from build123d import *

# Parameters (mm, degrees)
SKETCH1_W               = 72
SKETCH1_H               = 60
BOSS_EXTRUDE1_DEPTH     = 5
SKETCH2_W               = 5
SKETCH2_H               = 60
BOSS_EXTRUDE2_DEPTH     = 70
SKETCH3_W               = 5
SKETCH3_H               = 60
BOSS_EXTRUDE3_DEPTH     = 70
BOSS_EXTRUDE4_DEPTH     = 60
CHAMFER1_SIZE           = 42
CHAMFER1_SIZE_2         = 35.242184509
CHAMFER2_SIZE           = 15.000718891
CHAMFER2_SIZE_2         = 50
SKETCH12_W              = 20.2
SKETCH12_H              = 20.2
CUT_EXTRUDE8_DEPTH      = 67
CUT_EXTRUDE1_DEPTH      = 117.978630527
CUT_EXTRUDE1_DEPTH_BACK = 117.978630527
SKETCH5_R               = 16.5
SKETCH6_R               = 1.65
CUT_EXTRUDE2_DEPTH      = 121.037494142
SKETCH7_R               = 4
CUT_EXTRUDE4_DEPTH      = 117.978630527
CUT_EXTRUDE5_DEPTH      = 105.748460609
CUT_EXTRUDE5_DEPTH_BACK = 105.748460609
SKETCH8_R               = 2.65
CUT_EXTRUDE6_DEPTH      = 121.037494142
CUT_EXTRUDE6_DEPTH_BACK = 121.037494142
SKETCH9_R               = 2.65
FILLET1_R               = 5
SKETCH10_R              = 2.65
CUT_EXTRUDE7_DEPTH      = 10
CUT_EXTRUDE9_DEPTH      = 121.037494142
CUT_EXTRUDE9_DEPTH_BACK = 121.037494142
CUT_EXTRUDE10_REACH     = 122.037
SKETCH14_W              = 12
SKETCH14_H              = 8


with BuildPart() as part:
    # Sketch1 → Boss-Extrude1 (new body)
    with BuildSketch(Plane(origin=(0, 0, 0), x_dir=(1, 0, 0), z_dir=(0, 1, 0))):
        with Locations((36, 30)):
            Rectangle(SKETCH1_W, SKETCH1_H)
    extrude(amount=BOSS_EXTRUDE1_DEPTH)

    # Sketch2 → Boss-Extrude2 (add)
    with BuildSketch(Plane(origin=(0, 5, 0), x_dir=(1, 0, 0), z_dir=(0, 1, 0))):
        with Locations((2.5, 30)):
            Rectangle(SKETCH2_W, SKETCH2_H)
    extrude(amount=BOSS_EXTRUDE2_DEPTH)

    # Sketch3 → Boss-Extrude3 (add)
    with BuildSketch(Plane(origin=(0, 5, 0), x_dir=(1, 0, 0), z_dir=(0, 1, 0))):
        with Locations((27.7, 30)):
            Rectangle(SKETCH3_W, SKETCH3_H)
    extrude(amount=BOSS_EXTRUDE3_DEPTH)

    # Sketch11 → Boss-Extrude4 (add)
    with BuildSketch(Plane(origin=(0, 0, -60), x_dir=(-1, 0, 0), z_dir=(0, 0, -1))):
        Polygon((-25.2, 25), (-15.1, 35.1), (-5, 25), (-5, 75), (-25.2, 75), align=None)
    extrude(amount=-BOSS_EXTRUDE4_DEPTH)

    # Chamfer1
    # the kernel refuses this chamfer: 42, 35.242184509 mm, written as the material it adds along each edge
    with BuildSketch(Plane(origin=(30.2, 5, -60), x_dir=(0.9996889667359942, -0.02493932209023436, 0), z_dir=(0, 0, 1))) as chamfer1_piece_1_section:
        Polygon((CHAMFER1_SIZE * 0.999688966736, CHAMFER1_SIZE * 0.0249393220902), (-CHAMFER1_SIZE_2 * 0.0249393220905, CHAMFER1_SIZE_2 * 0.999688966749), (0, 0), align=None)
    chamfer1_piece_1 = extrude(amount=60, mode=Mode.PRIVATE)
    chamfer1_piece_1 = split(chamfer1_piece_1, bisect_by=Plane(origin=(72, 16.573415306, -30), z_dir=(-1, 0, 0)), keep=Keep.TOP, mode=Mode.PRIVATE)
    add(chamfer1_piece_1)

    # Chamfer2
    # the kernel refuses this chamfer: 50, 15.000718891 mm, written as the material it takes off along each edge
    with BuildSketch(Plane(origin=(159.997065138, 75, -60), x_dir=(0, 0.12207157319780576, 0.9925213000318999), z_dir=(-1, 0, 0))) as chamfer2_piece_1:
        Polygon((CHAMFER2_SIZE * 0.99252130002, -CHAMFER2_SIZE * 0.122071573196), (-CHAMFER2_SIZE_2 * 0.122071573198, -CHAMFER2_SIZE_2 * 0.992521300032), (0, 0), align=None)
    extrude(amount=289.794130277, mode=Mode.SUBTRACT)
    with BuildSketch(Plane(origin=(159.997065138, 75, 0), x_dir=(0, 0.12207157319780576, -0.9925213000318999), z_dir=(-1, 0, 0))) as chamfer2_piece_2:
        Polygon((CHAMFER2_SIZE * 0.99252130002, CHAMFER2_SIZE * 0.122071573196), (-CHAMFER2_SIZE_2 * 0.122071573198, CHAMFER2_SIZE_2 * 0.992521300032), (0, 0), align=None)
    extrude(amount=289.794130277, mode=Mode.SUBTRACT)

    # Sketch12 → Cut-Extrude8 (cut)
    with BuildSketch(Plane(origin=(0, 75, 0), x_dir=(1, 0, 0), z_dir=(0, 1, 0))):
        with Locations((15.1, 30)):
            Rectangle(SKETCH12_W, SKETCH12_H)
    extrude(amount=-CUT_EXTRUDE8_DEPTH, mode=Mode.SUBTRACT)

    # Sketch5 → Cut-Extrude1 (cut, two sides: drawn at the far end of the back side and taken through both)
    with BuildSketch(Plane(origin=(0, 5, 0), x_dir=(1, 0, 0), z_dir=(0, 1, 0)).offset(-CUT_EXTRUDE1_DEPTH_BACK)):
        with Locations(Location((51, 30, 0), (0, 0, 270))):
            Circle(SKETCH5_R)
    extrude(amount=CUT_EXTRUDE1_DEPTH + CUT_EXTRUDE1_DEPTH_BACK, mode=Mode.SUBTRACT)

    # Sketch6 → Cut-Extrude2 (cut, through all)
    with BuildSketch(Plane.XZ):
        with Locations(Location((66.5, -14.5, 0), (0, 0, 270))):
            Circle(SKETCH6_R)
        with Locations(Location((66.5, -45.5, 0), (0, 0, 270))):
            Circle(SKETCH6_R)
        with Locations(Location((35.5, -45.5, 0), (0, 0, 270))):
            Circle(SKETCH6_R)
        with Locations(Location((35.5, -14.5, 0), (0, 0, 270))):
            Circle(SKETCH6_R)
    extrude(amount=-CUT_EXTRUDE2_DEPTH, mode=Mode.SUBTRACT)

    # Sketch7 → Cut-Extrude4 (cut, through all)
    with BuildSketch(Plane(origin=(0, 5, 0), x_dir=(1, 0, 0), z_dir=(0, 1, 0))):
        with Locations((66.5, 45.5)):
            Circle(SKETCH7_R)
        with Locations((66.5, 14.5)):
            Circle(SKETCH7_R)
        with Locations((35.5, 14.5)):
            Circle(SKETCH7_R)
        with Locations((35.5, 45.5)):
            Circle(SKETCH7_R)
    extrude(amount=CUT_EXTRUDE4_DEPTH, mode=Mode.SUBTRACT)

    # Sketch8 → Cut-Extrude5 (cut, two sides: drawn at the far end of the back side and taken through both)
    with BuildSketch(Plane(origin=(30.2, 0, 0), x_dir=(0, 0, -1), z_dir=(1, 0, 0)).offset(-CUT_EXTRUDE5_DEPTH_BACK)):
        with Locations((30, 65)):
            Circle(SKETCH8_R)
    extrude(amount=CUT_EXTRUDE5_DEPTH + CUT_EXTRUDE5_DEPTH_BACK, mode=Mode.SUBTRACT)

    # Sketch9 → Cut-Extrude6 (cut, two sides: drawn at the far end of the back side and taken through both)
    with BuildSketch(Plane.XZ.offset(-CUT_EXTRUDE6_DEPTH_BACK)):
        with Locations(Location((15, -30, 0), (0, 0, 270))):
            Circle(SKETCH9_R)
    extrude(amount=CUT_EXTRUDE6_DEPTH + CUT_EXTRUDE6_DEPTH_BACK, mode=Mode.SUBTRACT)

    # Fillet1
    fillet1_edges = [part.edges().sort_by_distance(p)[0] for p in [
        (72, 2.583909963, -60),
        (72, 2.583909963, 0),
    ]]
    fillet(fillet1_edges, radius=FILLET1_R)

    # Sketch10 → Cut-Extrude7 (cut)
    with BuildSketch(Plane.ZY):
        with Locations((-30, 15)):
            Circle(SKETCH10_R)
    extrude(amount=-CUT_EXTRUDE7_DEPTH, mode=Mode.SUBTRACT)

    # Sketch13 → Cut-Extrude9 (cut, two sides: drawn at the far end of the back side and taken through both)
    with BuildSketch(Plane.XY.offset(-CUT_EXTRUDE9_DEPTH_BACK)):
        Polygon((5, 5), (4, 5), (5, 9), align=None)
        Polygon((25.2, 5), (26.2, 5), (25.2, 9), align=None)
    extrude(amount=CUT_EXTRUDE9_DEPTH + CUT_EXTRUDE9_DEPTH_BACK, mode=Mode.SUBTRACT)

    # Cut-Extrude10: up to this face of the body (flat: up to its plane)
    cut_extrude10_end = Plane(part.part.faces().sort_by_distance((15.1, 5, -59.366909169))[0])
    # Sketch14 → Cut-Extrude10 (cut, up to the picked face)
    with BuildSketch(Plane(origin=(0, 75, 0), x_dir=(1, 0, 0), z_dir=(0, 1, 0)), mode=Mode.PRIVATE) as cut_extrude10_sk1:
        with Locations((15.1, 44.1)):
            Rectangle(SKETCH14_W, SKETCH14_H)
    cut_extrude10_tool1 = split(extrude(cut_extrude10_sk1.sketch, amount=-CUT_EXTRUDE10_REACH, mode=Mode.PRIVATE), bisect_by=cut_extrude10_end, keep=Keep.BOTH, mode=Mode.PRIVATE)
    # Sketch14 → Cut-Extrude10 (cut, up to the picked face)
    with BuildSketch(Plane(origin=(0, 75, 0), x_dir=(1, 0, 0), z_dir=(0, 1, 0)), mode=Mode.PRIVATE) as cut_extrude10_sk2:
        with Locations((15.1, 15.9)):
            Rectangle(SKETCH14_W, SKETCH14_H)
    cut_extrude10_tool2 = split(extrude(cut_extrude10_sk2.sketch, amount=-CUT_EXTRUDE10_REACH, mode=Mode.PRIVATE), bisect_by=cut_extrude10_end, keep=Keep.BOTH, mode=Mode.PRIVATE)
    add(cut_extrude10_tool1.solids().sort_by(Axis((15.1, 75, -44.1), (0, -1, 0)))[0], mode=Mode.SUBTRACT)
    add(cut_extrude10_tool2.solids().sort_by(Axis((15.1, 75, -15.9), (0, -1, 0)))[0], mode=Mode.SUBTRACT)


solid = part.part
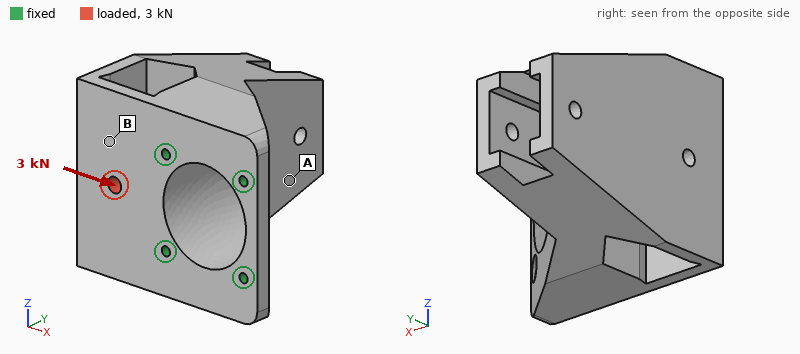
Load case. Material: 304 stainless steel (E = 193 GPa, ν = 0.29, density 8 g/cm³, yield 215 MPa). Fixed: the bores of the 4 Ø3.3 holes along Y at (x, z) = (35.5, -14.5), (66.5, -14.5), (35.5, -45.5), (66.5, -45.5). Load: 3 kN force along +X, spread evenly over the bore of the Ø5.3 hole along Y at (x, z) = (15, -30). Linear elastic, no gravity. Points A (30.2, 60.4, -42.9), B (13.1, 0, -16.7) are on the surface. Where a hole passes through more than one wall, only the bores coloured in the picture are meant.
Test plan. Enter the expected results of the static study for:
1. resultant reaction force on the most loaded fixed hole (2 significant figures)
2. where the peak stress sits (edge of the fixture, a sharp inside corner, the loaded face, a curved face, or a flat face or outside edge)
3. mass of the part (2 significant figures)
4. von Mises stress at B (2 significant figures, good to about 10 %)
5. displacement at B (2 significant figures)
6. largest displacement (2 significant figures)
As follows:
1.5 kN
the loaded face
720 g
7.5 MPa
1.7 µm
3.7 µm
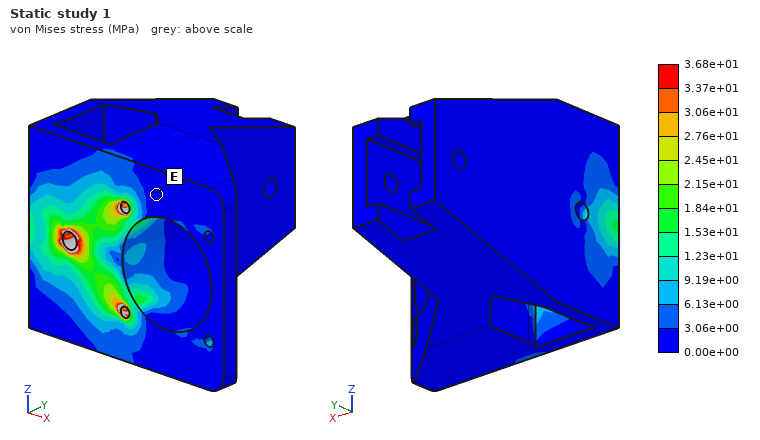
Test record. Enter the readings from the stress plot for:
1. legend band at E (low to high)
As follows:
0.00e+00 to 3.06e+00 MPa
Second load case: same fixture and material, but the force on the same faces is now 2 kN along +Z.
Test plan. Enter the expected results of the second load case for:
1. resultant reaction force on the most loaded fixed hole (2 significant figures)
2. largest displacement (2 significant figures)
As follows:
1.3 kN
3.9 µm
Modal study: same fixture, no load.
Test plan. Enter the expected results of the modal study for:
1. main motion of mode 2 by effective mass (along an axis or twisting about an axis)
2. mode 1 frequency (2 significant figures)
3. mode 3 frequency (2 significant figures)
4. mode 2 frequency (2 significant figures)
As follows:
along Z
2200 Hz
7100 Hz
3200 Hz
